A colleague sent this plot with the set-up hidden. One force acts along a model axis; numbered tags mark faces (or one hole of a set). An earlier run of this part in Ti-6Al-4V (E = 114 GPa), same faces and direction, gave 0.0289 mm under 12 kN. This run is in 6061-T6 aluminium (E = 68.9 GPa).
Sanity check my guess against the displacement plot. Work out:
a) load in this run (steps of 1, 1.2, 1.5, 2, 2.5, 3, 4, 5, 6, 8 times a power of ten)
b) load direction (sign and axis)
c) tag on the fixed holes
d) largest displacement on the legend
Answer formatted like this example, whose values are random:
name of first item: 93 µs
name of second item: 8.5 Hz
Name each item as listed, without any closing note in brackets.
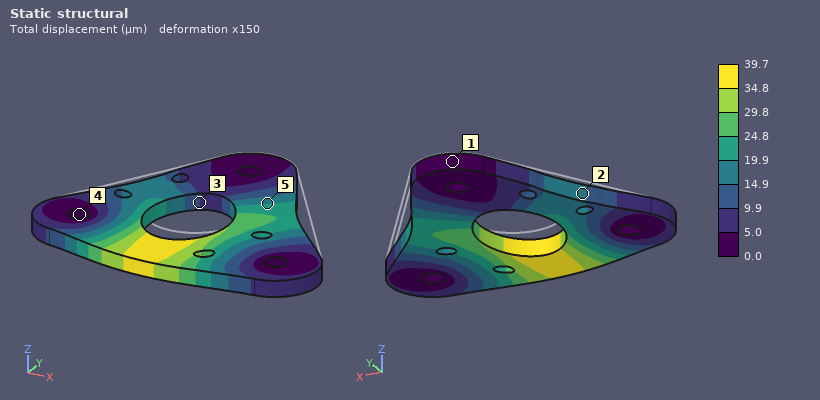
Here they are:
load in this run: 10 kN
load direction: -Y
tag on the fixed holes: 4
largest displacement on the legend: 39.7 µm
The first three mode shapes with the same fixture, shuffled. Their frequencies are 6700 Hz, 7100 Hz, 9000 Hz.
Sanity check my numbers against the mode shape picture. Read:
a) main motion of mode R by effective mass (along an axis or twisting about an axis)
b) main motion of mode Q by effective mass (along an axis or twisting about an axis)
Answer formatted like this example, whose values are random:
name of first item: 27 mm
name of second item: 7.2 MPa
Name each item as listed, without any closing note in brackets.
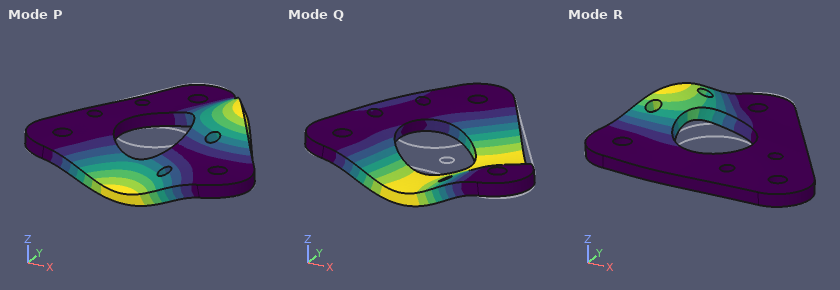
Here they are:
main motion of mode R by effective mass: along Z
main motion of mode Q by effective mass: along Z
